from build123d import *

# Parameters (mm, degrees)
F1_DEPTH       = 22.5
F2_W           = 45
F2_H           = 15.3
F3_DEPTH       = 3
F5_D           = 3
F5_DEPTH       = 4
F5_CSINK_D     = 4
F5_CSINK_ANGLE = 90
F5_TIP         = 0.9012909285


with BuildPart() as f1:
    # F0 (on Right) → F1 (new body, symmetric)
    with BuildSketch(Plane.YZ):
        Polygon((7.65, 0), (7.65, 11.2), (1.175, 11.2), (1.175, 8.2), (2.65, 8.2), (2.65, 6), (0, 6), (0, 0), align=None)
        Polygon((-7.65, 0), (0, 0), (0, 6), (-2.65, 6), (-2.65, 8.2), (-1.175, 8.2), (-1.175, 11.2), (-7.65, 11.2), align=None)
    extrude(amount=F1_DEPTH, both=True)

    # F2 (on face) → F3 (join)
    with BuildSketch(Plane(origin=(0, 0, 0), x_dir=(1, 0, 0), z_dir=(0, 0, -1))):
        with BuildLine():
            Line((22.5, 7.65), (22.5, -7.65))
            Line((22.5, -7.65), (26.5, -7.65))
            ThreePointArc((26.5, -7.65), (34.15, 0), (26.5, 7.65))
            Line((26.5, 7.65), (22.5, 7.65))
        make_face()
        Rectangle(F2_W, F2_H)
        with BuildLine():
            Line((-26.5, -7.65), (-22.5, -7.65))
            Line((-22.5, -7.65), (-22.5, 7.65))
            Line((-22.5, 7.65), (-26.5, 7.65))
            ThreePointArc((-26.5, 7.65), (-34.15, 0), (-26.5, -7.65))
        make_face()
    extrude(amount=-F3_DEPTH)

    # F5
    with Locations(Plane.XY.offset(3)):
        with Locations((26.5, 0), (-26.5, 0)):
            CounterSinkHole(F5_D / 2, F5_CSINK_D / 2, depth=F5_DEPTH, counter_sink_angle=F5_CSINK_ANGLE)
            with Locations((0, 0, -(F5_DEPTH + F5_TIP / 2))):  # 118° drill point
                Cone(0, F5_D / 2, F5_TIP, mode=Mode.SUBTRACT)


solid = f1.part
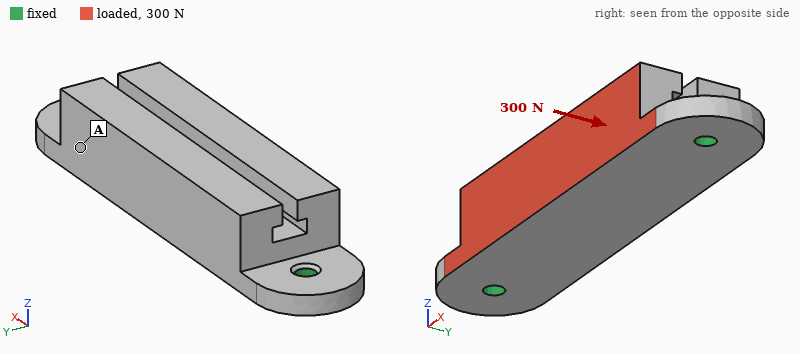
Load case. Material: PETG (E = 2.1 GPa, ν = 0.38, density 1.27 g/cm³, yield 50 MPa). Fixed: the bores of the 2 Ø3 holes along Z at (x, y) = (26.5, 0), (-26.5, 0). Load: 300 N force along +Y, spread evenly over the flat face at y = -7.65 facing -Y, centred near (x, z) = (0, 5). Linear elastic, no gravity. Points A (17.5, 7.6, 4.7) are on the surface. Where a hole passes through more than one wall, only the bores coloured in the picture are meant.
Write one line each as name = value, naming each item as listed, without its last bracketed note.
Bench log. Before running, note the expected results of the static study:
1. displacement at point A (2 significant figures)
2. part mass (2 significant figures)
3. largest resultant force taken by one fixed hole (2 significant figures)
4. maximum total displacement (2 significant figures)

displacement at point A = 0.27 mm
part mass = 9.8 g
largest resultant force taken by one fixed hole = 150 N
maximum total displacement = 0.52 mm
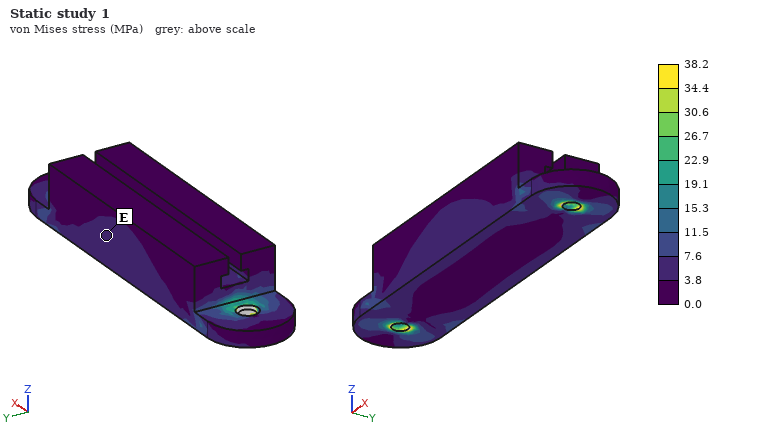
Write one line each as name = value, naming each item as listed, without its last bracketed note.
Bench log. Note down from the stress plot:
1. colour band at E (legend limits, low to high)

colour band at E = 3.8 to 7.6 MPa
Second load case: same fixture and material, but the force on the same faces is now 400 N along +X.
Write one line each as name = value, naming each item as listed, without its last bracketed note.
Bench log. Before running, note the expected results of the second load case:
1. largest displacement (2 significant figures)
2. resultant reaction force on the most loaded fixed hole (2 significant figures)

largest displacement = 56 µm
resultant reaction force on the most loaded fixed hole = 210 N
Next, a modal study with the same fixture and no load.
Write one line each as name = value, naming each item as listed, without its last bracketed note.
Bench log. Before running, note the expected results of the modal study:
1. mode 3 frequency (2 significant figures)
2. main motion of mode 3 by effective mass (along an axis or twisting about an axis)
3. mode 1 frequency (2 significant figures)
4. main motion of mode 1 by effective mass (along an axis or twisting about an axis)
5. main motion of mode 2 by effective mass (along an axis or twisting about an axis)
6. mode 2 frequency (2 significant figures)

mode 3 frequency = 3500 Hz
main motion of mode 3 by effective mass = along Y
mode 1 frequency = 1500 Hz
main motion of mode 1 by effective mass = along Y
main motion of mode 2 by effective mass = along Z
mode 2 frequency = 2500 Hz
